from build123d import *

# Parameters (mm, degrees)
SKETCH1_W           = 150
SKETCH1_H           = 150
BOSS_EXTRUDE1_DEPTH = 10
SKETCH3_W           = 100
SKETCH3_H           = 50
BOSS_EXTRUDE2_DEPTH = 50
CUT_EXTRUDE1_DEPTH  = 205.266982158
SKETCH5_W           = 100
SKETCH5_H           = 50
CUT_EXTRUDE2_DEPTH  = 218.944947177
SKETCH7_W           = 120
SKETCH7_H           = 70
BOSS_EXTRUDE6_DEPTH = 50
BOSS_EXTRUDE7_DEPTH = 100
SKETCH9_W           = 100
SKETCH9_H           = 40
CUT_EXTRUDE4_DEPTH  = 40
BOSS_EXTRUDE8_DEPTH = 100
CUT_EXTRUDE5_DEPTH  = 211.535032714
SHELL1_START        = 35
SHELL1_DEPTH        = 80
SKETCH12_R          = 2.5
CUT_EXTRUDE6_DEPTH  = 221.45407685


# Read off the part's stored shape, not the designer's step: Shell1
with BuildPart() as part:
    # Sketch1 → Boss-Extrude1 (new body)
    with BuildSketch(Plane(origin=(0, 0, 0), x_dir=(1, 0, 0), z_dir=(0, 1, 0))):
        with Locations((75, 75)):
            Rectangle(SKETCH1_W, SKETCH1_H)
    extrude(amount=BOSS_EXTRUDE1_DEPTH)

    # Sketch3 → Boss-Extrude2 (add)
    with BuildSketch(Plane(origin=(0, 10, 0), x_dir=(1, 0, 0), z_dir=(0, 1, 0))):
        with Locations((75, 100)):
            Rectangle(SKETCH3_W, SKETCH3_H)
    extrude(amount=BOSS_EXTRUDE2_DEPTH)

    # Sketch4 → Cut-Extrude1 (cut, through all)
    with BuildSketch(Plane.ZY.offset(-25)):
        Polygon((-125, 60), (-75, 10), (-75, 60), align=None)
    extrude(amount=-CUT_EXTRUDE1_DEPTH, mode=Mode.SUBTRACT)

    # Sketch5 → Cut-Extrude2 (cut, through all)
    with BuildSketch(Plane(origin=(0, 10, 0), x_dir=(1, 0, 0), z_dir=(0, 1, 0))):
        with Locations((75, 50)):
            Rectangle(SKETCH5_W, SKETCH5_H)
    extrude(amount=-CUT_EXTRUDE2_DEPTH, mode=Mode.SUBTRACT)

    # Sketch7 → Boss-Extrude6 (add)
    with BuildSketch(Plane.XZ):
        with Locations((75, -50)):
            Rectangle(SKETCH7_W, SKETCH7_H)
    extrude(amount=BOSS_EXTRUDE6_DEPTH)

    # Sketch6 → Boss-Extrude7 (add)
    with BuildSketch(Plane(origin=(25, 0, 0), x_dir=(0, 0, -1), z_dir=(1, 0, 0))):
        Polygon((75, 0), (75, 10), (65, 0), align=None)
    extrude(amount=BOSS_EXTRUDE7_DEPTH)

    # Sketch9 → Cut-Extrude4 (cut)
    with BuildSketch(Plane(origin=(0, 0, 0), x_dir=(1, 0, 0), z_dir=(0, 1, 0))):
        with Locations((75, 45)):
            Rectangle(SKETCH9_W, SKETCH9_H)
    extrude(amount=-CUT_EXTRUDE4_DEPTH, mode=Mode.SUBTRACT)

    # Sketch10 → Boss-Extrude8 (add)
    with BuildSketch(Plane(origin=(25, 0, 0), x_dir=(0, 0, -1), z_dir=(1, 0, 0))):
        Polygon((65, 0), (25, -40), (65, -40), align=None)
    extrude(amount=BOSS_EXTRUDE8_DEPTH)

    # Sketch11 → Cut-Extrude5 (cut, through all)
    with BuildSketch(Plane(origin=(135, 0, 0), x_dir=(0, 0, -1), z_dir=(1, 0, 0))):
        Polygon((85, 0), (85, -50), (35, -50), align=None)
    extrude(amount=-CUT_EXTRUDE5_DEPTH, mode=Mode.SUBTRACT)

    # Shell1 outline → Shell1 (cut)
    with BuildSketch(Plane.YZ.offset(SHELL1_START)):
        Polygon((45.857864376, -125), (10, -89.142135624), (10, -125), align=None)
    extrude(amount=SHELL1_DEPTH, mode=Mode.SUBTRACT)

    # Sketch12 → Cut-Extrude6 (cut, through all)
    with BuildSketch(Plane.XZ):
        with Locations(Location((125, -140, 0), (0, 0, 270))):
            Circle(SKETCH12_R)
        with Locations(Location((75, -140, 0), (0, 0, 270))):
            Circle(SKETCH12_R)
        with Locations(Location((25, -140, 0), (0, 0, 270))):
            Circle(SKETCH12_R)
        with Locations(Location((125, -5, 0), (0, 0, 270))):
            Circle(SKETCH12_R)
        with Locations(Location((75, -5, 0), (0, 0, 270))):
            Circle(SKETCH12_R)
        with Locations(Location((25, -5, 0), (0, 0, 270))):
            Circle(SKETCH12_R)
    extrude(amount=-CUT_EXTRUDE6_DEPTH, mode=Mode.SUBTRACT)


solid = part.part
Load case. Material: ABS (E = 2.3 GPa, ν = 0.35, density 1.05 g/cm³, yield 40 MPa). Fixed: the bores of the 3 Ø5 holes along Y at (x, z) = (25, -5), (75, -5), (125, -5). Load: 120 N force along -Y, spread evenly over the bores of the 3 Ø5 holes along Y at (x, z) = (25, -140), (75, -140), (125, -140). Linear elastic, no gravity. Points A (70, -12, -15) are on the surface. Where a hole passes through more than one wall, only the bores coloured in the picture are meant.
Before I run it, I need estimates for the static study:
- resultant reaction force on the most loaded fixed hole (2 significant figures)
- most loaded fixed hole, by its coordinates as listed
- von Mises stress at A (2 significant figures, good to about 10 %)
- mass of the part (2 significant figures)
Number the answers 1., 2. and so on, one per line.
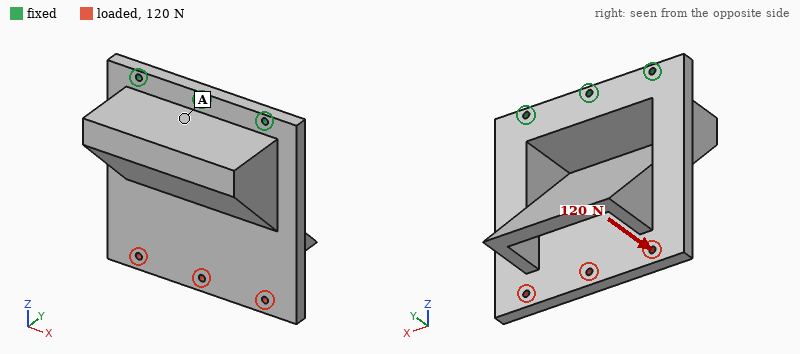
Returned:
1. 150 N
2. (75, -5)
3. 1.9 MPa
4. 460 g
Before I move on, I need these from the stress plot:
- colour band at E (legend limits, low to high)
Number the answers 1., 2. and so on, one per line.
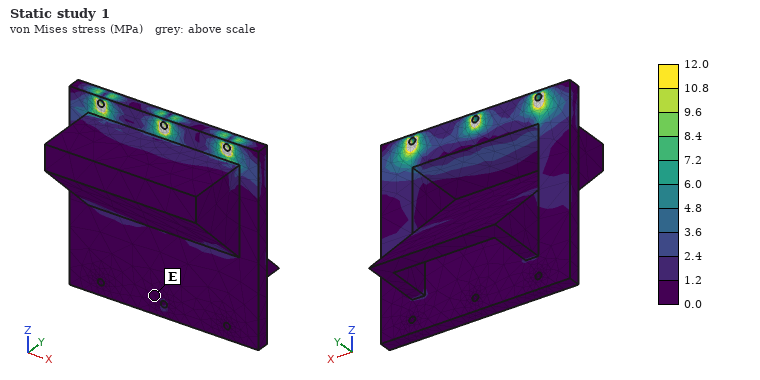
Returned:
1. 0.0 to 1.2 MPa
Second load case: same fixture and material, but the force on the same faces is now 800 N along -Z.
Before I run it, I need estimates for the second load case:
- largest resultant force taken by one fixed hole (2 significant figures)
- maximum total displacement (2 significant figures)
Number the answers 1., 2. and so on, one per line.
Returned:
1. 420 N
2. 0.32 mm
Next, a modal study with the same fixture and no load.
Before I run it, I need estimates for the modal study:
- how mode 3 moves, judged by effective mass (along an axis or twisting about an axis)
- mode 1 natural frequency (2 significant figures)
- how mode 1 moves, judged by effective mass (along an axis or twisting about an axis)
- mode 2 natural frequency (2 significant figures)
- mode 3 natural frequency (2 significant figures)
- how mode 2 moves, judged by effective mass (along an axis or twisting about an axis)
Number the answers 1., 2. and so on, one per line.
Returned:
1. along X
2. 93 Hz
3. along Y
4. 300 Hz
5. 600 Hz
6. along X
